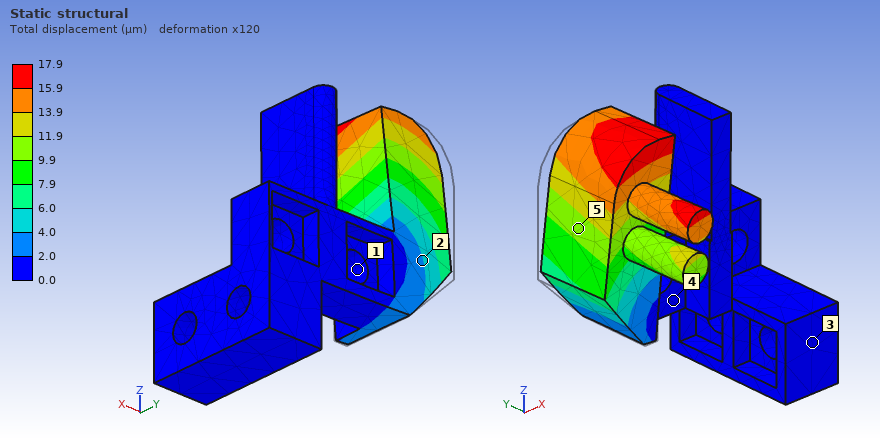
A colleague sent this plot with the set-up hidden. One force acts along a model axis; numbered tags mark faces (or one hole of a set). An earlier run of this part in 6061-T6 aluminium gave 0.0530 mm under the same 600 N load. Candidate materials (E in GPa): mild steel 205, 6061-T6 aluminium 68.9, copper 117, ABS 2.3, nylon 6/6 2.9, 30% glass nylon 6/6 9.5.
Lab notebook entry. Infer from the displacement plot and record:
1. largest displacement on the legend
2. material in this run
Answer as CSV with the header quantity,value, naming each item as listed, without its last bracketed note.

quantity,value
largest displacement on the legend,17.9 µm
material in this run,mild steel
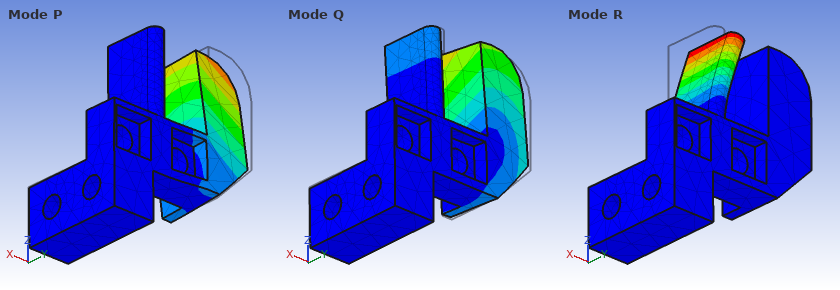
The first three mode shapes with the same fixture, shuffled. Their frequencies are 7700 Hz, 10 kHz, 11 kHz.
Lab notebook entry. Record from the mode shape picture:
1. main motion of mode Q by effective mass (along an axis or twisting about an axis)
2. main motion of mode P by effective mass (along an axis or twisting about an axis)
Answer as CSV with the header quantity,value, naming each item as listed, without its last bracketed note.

quantity,value
main motion of mode Q by effective mass,along X
main motion of mode P by effective mass,along Y
